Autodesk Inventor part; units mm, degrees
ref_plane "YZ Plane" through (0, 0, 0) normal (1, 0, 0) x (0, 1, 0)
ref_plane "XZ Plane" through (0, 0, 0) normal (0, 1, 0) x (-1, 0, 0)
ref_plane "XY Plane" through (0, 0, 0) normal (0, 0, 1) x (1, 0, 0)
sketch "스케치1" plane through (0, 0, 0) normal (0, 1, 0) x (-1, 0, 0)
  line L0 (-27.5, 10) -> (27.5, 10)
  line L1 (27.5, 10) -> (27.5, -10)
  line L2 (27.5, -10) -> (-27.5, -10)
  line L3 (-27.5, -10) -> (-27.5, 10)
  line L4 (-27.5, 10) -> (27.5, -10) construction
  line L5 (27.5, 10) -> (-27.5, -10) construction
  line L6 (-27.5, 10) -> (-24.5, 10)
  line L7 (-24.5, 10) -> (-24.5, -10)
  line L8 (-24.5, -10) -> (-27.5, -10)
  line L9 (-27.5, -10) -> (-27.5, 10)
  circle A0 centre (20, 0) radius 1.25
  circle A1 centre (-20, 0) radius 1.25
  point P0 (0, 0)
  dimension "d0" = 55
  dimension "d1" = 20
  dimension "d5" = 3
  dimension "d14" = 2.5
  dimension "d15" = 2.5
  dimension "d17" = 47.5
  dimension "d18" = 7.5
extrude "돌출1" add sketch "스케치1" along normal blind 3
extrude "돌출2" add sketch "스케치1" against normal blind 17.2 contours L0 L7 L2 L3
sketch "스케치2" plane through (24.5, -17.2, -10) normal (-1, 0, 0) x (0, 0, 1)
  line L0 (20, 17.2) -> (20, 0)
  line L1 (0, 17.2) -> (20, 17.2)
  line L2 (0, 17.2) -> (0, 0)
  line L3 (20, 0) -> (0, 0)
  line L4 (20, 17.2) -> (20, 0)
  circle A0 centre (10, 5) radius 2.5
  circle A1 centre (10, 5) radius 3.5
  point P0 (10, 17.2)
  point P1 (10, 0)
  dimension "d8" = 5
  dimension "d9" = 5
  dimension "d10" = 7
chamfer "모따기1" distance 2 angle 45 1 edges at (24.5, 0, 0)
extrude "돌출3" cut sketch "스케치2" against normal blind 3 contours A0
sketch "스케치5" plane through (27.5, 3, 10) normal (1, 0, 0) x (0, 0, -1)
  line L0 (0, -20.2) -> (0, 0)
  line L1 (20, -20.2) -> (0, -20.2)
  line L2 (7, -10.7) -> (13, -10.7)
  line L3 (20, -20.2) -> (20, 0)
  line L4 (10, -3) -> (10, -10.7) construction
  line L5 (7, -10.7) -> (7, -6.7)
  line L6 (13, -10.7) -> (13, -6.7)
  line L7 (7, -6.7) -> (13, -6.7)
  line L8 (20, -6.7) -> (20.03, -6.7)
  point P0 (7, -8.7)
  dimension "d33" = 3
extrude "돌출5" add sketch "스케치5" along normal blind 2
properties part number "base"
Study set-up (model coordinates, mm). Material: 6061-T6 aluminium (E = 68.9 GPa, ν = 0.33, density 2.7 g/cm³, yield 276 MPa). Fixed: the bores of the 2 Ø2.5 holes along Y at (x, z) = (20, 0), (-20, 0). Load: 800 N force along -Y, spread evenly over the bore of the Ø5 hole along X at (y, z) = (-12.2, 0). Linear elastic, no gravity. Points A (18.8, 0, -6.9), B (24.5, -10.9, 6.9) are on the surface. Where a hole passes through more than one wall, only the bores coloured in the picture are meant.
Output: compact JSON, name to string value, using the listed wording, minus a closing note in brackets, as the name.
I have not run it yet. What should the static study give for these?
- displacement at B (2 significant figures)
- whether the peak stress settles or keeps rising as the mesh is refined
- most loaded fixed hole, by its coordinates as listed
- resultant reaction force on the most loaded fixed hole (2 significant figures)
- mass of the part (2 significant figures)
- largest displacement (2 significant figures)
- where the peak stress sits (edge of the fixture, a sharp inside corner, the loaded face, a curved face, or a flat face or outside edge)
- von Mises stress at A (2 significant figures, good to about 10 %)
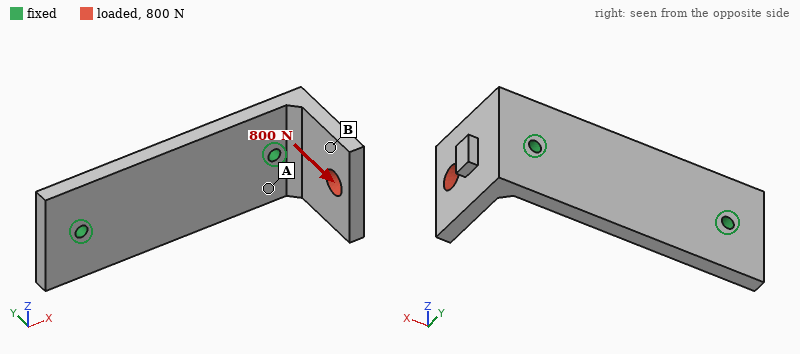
{"displacement at B": "0.076 mm", "whether the peak stress settles or keeps rising as the mesh is refined": "keeps rising", "most loaded fixed hole, by its coordinates as listed": "(20, 0)", "resultant reaction force on the most loaded fixed hole": "820 N", "mass of the part": "12 g", "largest displacement": "0.12 mm", "where the peak stress sits": "edge of the fixture", "von Mises stress at A": "49 MPa"}
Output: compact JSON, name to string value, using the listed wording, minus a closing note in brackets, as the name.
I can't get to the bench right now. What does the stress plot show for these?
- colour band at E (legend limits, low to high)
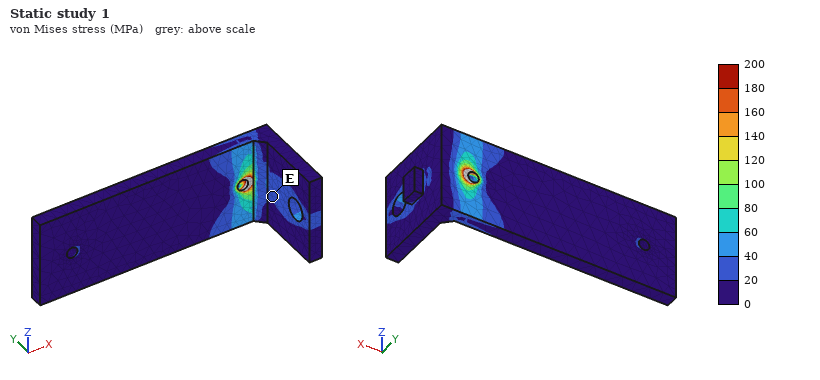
{"colour band at E": "20 to 40 MPa"}
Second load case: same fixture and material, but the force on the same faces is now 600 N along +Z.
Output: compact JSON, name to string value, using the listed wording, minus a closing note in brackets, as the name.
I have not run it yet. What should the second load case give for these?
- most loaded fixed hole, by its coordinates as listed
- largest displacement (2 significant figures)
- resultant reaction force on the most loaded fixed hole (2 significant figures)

{"most loaded fixed hole, by its coordinates as listed": "(20, 0)", "largest displacement": "0.22 mm", "resultant reaction force on the most loaded fixed hole": "670 N"}
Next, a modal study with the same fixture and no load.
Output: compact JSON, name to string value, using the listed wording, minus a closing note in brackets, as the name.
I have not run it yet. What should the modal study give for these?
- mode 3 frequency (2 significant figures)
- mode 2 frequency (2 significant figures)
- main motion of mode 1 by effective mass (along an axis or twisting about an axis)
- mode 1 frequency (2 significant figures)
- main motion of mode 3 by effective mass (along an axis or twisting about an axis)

{"mode 3 frequency": "8500 Hz", "mode 2 frequency": "6500 Hz", "main motion of mode 1 by effective mass": "along X", "mode 1 frequency": "5200 Hz", "main motion of mode 3 by effective mass": "along Y"}
